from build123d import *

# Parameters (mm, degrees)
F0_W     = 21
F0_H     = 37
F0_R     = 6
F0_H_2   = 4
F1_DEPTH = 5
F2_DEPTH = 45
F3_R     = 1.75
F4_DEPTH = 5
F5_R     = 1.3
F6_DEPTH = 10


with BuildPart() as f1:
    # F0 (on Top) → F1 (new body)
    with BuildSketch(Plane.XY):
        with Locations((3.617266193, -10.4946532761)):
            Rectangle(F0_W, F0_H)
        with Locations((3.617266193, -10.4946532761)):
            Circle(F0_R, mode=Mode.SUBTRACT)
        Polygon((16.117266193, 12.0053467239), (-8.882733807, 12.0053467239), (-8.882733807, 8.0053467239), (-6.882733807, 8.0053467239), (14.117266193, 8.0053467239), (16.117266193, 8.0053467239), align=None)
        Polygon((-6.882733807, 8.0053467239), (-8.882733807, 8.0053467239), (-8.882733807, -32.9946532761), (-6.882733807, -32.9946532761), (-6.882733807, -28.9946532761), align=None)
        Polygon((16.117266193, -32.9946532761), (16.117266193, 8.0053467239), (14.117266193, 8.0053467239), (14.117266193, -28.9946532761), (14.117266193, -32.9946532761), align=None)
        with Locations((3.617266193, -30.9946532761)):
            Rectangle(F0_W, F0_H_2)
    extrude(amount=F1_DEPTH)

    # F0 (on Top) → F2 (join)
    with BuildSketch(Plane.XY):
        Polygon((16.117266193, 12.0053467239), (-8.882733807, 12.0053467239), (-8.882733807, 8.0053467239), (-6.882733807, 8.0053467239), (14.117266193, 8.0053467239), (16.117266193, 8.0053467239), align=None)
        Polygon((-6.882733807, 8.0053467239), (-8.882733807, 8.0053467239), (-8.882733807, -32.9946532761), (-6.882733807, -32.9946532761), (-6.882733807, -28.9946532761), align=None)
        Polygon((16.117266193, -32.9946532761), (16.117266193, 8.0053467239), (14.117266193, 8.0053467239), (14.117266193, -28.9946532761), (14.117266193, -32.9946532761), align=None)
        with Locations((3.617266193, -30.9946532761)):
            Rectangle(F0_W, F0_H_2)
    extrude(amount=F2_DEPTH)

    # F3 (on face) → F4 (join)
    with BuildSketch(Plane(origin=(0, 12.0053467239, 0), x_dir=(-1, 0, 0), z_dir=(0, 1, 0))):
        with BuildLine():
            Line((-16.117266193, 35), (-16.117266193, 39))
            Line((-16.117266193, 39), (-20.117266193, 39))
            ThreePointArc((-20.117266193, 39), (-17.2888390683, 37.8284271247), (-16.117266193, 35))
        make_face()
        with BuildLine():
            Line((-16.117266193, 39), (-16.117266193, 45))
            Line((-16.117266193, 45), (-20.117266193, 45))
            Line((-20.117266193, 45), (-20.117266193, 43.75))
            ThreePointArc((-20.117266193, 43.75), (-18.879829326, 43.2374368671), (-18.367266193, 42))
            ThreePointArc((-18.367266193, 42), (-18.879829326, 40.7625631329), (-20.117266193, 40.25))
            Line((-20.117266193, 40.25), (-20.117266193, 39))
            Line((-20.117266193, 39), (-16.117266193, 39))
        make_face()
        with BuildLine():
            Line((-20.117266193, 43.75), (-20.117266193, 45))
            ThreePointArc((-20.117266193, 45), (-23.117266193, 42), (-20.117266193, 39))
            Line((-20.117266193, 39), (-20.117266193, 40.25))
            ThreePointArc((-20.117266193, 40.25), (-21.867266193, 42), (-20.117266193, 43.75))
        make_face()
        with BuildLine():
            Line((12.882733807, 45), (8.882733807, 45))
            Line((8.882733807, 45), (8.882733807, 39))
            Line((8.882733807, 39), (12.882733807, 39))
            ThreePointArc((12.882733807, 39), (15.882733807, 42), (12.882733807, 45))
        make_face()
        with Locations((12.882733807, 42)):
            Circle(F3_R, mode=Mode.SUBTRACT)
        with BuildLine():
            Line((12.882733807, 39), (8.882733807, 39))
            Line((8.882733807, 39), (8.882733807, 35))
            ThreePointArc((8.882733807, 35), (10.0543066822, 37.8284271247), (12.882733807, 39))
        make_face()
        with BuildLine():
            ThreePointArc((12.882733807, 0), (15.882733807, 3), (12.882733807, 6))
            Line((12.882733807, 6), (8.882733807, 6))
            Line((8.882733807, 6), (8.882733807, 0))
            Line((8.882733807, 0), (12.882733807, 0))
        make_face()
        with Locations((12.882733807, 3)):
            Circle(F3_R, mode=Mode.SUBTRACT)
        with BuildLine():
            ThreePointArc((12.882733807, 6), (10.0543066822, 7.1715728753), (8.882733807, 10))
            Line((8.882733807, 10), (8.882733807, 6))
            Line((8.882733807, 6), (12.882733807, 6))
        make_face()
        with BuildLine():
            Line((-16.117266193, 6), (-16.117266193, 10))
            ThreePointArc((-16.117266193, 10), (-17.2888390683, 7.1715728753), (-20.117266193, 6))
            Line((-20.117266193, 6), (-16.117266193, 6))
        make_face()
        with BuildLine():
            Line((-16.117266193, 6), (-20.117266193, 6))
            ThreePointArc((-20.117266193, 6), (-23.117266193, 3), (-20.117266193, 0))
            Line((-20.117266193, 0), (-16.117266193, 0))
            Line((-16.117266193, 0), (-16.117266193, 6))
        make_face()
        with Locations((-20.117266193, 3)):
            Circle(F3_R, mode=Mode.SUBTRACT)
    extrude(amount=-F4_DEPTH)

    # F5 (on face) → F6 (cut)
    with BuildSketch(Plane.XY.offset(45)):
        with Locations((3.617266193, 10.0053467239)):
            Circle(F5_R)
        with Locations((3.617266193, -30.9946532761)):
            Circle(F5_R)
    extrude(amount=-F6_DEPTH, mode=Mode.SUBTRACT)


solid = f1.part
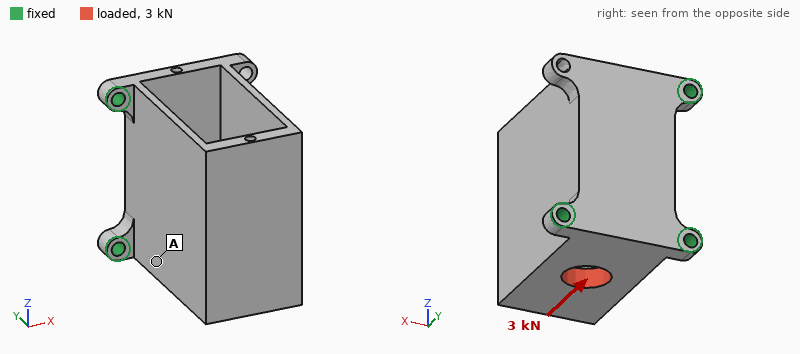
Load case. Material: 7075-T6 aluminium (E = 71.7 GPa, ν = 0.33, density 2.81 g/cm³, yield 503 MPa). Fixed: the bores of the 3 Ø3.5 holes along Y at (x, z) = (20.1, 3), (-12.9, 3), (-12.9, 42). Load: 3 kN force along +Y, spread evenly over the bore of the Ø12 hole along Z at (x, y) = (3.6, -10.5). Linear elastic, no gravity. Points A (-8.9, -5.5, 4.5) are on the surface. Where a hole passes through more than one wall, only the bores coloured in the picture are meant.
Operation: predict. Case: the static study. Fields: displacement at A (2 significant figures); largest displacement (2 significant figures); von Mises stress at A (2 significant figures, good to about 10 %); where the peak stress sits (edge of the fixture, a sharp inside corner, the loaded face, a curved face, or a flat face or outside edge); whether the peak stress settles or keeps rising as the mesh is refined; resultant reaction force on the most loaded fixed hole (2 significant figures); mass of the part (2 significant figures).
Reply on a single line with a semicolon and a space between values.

17 µm; 33 µm; 17 MPa; edge of the fixture; keeps rising; 1.6 kN; 55 g
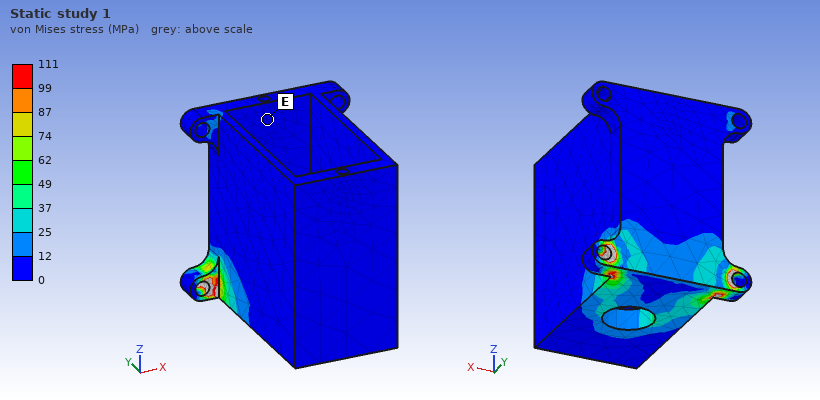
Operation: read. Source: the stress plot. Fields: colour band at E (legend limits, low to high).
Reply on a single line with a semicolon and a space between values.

0 to 12 MPa
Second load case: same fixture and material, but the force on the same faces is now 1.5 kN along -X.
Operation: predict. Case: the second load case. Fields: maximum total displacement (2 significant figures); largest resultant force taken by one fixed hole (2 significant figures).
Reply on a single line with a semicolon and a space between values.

60 µm; 1.3 kN
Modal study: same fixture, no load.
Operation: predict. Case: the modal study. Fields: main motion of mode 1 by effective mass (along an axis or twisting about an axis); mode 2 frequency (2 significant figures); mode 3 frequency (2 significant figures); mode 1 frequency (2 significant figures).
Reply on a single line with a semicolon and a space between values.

along X; 3500 Hz; 6800 Hz; 2100 Hz
